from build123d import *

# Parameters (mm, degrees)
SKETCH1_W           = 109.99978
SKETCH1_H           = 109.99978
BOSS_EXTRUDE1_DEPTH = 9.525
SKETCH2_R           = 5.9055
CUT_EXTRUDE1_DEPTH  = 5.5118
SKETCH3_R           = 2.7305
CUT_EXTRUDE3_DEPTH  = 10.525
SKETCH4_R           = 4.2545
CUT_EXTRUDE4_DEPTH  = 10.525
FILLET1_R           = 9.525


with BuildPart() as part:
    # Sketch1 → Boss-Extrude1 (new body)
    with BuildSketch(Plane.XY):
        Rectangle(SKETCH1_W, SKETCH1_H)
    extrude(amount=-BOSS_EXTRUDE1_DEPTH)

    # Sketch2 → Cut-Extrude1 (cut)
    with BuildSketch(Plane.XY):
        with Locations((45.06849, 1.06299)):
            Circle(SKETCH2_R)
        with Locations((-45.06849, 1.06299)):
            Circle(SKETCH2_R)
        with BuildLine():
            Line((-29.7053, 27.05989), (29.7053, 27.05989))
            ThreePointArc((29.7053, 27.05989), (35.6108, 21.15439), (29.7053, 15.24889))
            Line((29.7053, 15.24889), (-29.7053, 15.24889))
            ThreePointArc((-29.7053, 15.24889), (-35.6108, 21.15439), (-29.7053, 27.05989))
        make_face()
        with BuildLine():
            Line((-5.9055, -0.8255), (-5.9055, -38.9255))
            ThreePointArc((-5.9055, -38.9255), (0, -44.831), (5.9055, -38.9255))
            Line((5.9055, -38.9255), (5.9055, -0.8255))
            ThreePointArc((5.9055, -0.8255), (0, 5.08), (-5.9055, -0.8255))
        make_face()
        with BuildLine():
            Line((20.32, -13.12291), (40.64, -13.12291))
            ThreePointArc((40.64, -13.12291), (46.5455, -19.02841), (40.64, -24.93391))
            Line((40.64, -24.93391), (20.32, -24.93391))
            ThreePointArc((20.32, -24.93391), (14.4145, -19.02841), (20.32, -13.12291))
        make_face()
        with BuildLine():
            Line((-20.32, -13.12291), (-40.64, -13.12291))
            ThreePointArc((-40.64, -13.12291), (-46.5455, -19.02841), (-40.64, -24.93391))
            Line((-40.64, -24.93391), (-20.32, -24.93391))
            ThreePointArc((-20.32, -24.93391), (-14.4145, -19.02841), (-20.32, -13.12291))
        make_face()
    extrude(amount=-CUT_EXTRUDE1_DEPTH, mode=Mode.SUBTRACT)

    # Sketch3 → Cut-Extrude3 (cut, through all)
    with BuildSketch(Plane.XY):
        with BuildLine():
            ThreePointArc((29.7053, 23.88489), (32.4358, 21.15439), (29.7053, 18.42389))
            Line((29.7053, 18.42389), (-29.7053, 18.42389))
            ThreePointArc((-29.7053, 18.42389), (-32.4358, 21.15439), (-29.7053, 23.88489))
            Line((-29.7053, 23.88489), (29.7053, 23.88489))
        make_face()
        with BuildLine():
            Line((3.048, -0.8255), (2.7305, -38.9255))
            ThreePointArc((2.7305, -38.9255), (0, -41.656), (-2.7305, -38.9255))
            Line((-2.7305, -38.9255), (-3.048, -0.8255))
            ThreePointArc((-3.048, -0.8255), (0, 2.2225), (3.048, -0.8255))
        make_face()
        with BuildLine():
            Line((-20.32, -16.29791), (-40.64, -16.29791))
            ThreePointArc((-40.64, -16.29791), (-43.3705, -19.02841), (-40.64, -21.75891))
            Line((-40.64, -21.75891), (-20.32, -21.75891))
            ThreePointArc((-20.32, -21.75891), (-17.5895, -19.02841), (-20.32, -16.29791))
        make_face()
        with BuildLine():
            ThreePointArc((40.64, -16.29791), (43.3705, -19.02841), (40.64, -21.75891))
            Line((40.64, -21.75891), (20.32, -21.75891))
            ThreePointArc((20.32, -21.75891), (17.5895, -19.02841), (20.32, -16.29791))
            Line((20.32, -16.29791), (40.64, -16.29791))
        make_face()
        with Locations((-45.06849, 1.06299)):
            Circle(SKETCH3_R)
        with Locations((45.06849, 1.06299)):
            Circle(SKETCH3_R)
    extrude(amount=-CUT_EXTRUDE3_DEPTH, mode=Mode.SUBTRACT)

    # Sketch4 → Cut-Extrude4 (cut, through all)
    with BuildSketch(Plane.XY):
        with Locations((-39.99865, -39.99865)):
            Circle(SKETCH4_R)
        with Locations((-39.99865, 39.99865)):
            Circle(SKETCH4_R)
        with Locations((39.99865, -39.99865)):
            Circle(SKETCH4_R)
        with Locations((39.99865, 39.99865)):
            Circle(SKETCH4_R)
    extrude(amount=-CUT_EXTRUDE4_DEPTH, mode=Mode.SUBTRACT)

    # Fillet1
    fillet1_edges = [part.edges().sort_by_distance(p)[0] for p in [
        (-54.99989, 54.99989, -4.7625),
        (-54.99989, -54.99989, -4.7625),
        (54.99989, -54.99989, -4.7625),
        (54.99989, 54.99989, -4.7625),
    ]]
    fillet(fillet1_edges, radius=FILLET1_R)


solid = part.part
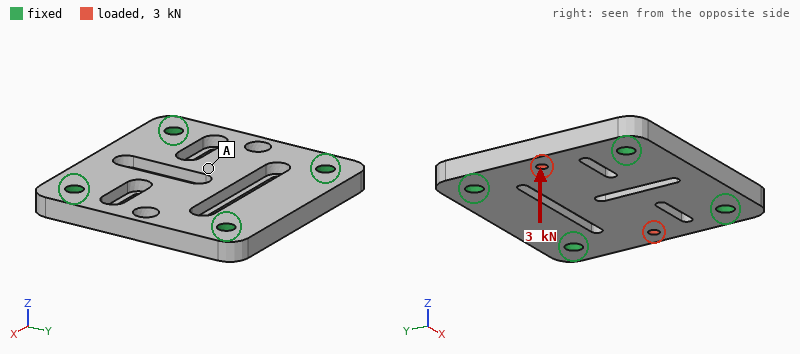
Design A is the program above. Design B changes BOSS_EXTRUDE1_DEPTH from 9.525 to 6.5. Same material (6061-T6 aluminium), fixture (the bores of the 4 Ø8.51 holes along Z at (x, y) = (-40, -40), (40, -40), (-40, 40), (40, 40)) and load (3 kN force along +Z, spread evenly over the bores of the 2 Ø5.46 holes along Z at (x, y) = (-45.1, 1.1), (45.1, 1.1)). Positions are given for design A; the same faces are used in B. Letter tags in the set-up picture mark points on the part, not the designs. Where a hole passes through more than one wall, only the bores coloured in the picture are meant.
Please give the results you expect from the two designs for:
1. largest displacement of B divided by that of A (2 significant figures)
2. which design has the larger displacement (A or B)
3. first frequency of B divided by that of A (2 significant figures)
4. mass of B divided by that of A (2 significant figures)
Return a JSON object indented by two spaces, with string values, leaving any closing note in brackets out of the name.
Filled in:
{
  "largest displacement of B divided by that of A": "4.7",
  "which design has the larger displacement": "B",
  "first frequency of B divided by that of A": "0.74",
  "mass of B divided by that of A": "0.66"
}
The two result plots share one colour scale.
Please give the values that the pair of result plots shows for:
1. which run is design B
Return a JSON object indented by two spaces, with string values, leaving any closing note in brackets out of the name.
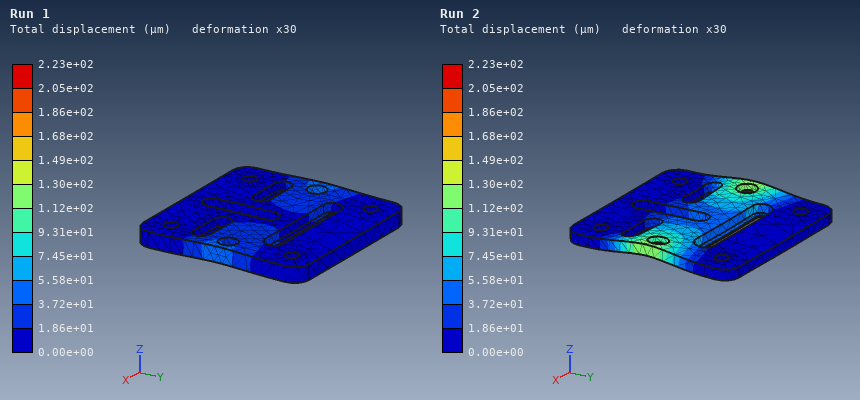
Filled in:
{
  "which run is design B": "Run 2"
}
